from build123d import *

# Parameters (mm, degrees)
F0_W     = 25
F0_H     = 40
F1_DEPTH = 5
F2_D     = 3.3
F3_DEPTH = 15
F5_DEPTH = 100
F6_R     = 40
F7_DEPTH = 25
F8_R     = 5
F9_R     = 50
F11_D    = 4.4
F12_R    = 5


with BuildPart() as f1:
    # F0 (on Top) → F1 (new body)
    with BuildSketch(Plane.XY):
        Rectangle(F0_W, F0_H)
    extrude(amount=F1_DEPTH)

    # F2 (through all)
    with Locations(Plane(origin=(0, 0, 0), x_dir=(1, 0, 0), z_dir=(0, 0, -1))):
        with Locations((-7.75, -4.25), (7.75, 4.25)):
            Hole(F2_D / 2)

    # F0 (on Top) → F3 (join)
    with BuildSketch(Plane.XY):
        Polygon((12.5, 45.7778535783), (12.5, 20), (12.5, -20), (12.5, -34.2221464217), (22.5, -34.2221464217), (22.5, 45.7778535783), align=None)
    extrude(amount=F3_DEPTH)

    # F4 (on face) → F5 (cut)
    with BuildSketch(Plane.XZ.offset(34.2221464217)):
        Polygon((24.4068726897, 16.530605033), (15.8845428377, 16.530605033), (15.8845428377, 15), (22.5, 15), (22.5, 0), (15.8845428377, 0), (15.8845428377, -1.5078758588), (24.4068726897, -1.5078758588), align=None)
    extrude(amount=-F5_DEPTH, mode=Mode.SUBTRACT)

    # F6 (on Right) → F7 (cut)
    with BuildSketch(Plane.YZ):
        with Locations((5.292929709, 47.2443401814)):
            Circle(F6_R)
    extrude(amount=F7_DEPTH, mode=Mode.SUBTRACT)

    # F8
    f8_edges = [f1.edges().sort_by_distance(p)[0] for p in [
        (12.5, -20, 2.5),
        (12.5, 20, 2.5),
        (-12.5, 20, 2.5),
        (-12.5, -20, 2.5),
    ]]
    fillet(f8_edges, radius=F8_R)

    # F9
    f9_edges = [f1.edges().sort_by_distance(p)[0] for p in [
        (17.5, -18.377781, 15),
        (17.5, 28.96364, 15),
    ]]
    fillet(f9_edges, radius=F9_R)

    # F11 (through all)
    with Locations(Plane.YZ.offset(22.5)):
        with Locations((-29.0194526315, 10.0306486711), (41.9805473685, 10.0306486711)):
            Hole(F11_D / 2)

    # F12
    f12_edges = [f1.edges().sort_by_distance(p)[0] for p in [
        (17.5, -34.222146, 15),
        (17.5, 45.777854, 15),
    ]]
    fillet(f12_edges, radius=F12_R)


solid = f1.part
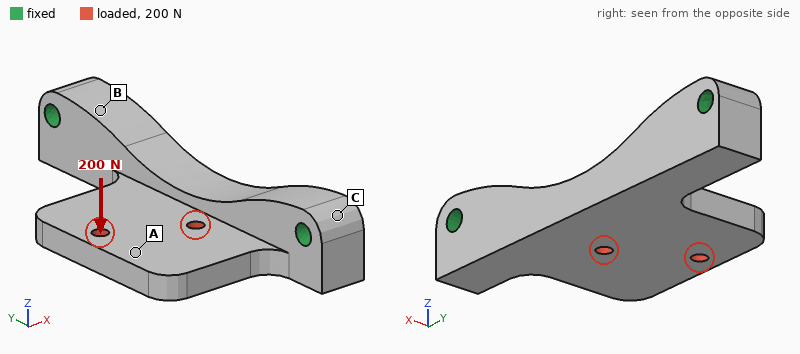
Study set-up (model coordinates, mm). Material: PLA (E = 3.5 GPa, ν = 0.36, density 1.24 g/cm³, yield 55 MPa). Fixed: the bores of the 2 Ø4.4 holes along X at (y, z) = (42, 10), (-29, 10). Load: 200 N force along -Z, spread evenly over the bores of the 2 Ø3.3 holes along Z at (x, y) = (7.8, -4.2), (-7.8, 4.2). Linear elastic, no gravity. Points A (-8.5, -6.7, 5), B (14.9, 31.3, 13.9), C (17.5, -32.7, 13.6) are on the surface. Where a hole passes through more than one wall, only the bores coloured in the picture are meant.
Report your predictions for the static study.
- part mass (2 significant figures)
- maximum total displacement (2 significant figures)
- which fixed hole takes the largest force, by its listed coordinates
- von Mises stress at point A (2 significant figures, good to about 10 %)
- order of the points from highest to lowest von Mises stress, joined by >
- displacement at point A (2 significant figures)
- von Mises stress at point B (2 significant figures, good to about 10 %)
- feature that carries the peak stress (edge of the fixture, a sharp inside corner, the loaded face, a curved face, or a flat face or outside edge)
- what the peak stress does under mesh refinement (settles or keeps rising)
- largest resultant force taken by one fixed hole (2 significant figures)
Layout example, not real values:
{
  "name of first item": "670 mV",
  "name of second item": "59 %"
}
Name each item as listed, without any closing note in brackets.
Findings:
{
  "part mass": "17 g",
  "maximum total displacement": "0.92 mm",
  "which fixed hole takes the largest force, by its listed coordinates": "(-29, 10)",
  "von Mises stress at point A": "4.1 MPa",
  "order of the points from highest to lowest von Mises stress, joined by >": "B > A > C",
  "displacement at point A": "0.69 mm",
  "von Mises stress at point B": "6.6 MPa",
  "feature that carries the peak stress": "edge of the fixture",
  "what the peak stress does under mesh refinement": "keeps rising",
  "largest resultant force taken by one fixed hole": "200 N"
}
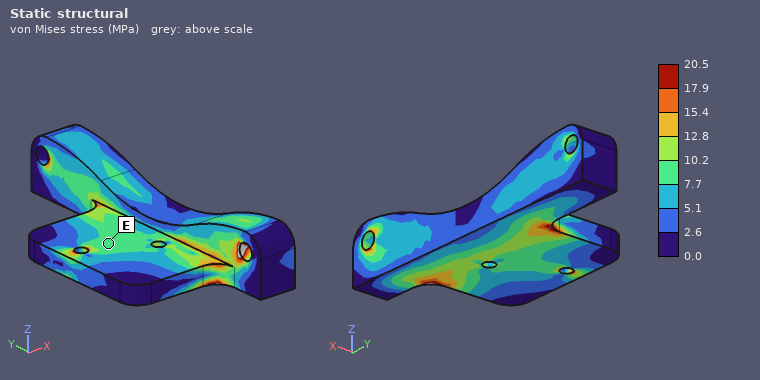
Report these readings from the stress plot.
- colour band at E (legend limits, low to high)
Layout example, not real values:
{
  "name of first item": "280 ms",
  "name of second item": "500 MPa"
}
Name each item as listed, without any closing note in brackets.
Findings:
{
  "colour band at E": "7.7 to 10.2 MPa"
}
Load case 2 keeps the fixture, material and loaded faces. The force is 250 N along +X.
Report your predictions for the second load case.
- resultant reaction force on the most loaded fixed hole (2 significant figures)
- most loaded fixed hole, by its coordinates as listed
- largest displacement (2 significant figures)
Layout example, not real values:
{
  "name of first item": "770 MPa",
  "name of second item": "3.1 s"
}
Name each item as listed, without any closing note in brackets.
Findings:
{
  "resultant reaction force on the most loaded fixed hole": "150 N",
  "most loaded fixed hole, by its coordinates as listed": "(-29, 10)",
  "largest displacement": "0.15 mm"
}
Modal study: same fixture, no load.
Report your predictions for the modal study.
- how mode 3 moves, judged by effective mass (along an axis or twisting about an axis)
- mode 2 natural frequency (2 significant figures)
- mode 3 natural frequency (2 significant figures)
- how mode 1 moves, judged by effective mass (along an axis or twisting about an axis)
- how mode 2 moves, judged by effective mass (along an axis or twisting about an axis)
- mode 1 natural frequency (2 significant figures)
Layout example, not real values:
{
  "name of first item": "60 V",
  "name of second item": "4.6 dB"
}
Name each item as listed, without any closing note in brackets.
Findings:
{
  "how mode 3 moves, judged by effective mass": "along X",
  "mode 2 natural frequency": "2800 Hz",
  "mode 3 natural frequency": "3000 Hz",
  "how mode 1 moves, judged by effective mass": "along Z",
  "how mode 2 moves, judged by effective mass": "along X",
  "mode 1 natural frequency": "1200 Hz"
}
